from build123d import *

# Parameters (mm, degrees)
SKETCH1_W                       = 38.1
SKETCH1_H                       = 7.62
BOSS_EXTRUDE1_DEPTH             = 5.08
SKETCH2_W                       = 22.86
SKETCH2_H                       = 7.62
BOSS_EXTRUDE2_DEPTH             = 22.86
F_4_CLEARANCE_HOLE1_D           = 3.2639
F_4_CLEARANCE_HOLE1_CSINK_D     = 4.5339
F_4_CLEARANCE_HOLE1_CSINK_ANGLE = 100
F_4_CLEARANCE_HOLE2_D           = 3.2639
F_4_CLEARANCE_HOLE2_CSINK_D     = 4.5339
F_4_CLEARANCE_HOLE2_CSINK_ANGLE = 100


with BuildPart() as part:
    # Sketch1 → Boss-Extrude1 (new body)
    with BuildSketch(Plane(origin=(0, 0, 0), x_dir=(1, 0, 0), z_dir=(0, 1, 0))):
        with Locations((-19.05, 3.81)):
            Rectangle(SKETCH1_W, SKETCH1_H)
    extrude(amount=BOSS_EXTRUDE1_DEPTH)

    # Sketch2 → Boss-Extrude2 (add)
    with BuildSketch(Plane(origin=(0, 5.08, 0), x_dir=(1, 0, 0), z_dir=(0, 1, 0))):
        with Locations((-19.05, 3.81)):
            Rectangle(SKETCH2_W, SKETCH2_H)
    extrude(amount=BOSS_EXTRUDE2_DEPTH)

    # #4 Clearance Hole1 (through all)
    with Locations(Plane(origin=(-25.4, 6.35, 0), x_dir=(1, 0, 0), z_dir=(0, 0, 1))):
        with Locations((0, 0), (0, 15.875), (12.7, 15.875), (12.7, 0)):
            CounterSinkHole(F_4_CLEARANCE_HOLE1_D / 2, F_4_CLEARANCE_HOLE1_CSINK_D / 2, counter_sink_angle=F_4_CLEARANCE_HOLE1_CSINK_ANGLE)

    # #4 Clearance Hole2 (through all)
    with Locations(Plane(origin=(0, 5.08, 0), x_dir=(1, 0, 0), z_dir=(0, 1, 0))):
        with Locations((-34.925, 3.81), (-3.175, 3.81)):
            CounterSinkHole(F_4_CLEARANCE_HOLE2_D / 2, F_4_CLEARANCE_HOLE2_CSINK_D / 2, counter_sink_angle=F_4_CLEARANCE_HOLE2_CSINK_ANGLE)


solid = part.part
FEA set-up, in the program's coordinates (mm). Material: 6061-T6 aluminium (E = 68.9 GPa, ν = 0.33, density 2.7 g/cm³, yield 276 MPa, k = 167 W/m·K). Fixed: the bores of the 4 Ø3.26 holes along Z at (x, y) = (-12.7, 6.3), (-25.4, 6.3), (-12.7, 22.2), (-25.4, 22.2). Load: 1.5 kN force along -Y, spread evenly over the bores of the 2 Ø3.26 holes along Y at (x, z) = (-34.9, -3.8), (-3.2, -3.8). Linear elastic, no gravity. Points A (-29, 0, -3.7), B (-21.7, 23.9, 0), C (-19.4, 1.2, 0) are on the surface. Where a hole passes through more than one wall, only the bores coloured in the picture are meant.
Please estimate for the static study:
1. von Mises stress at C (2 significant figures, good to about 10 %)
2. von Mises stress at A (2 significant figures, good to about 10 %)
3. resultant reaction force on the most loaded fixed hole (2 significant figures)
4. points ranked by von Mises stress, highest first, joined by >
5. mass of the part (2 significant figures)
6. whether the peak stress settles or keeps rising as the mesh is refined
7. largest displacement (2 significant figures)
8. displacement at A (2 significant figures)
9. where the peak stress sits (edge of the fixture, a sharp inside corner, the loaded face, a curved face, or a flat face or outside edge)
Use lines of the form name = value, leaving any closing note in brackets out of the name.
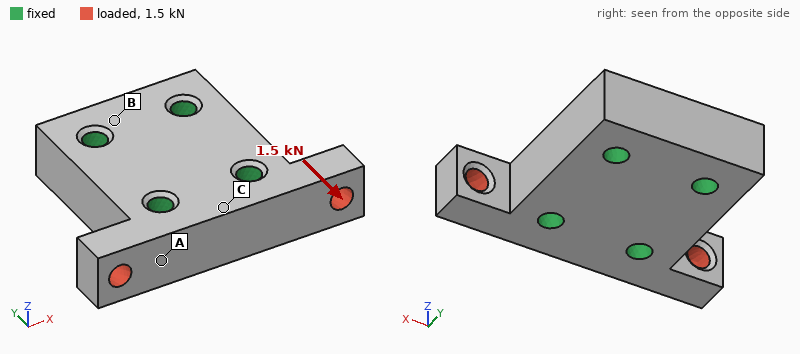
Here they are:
von Mises stress at C = 22 MPa
von Mises stress at A = 83 MPa
resultant reaction force on the most loaded fixed hole = 730 N
points ranked by von Mises stress, highest first, joined by > = A > C > B
mass of the part = 14 g
whether the peak stress settles or keeps rising as the mesh is refined = keeps rising
largest displacement = 39 µm
displacement at A = 7.6 µm
where the peak stress sits = edge of the fixture
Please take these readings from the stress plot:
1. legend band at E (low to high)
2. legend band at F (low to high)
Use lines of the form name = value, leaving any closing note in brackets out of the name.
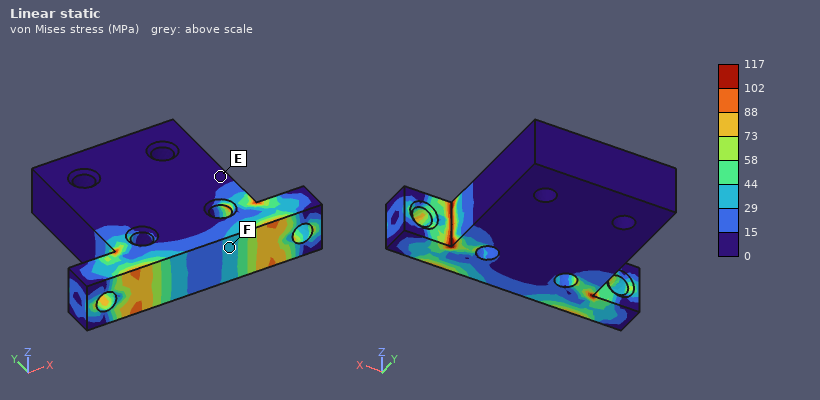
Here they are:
legend band at E = 0 to 15 MPa
legend band at F = 29 to 44 MPa
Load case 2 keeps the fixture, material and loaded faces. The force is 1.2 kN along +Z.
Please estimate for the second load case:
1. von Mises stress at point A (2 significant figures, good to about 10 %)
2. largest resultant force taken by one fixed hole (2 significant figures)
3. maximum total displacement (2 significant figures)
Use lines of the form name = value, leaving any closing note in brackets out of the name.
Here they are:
von Mises stress at point A = 23 MPa
largest resultant force taken by one fixed hole = 620 N
maximum total displacement = 29 µm
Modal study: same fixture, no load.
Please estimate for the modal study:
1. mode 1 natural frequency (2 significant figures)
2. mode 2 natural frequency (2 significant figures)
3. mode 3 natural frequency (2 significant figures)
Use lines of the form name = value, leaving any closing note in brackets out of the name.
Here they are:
mode 1 natural frequency = 33 kHz
mode 2 natural frequency = 34 kHz
mode 3 natural frequency = 34 kHz
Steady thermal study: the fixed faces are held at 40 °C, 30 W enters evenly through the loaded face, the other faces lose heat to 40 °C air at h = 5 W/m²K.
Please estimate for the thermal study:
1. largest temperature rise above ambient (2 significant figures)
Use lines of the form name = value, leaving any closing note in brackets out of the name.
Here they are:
largest temperature rise above ambient = 25 K
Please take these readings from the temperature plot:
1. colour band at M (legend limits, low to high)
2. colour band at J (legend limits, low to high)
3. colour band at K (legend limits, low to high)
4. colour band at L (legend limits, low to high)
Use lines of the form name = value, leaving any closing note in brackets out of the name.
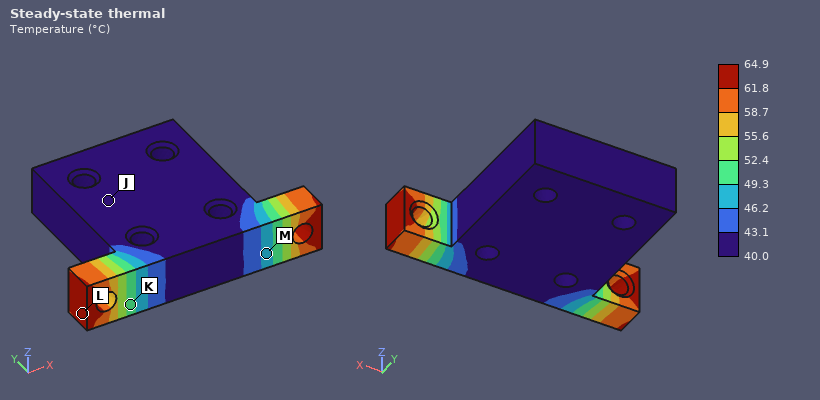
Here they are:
colour band at M = 46.2 to 49.3 °C
colour band at J = 40.0 to 43.1 °C
colour band at K = 49.3 to 52.4 °C
colour band at L = 61.8 to 64.9 °C
